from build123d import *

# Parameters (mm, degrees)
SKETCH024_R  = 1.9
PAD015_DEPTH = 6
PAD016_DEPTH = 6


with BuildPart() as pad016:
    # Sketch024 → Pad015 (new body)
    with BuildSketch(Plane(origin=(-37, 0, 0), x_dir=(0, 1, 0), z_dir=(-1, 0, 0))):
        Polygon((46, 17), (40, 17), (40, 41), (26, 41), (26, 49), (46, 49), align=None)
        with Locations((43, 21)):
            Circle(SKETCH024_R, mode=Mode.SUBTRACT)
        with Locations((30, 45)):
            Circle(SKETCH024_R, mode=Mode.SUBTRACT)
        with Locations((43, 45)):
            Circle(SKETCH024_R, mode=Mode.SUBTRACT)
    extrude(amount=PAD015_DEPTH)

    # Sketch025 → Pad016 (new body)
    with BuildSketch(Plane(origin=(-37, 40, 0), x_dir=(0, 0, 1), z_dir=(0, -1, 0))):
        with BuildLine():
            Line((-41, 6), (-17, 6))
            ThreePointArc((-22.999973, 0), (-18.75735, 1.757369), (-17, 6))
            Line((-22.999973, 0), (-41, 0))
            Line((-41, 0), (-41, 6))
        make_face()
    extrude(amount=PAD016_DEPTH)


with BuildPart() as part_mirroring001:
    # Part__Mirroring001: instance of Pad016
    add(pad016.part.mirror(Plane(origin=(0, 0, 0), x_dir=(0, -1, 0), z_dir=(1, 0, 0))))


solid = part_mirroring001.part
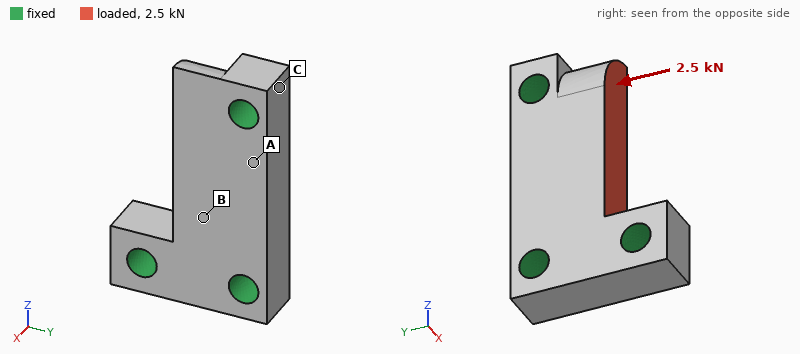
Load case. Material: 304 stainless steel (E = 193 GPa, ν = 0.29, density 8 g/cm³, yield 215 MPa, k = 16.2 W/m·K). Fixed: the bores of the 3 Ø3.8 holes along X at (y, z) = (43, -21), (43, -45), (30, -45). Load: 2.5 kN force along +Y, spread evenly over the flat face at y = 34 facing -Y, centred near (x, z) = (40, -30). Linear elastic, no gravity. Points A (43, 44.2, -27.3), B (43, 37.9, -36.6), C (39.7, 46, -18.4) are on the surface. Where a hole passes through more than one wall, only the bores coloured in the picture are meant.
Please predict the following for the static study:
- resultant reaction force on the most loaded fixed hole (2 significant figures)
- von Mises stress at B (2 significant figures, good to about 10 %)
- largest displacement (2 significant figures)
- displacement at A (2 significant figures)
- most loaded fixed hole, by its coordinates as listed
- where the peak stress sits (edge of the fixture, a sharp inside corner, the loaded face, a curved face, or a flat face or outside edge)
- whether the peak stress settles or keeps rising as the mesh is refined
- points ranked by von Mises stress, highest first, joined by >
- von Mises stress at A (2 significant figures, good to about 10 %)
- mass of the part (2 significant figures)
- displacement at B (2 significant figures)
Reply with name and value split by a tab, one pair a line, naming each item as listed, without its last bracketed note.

resultant reaction force on the most loaded fixed hole	1.5 kN
von Mises stress at B	22 MPa
largest displacement	2.3 µm
displacement at A	1.4 µm
most loaded fixed hole, by its coordinates as listed	(43, -21)
where the peak stress sits	edge of the fixture
whether the peak stress settles or keeps rising as the mesh is refined	keeps rising
points ranked by von Mises stress, highest first, joined by >	B > A > C
von Mises stress at A	12 MPa
mass of the part	20 g
displacement at B	1.7 µm
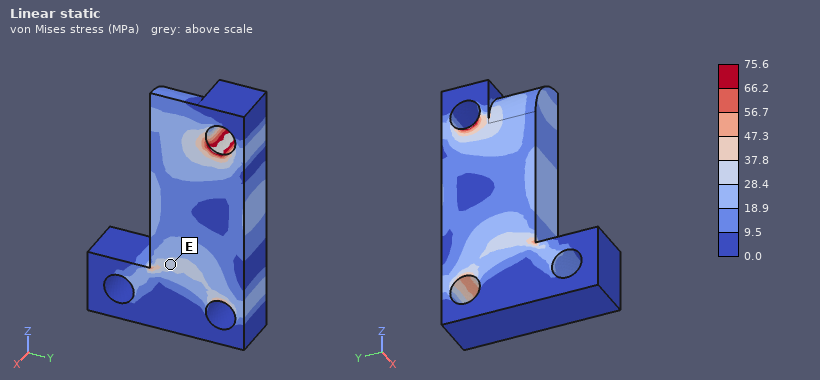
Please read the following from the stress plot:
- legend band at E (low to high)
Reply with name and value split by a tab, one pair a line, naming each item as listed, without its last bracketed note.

legend band at E	28.4 to 37.8 MPa
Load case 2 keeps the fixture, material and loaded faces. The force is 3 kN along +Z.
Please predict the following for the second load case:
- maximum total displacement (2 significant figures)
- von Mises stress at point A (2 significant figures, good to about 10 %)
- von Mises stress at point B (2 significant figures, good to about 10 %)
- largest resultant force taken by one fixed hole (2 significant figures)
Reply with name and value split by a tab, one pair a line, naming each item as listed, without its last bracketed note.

maximum total displacement	5.2 µm
von Mises stress at point A	13 MPa
von Mises stress at point B	33 MPa
largest resultant force taken by one fixed hole	1.6 kN
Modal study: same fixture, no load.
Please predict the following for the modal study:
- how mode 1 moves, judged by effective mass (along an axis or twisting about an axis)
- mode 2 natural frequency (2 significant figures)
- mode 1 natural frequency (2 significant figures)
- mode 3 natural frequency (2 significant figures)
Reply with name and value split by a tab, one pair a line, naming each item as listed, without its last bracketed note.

how mode 1 moves, judged by effective mass	along X
mode 2 natural frequency	52 kHz
mode 1 natural frequency	37 kHz
mode 3 natural frequency	52 kHz
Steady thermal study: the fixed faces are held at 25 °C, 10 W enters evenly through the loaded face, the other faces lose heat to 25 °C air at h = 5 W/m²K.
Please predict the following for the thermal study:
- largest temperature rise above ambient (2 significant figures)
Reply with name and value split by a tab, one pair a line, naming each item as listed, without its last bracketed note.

largest temperature rise above ambient	48 K
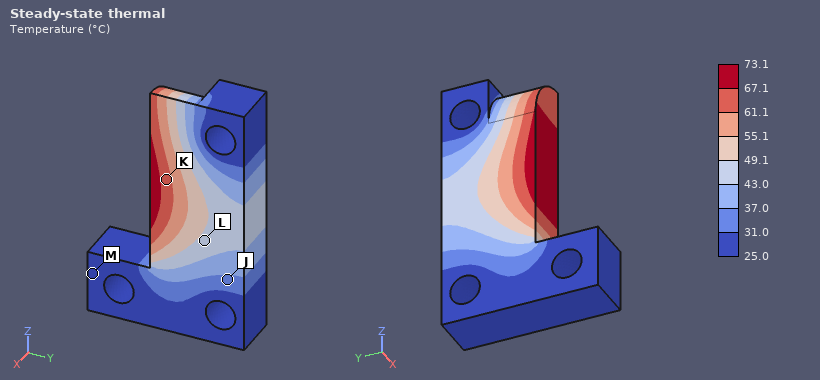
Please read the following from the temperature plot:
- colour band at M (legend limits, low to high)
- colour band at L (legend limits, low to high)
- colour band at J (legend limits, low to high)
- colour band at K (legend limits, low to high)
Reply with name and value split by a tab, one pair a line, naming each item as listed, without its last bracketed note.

colour band at M	25.0 to 31.0 °C
colour band at L	43.0 to 49.1 °C
colour band at J	31.0 to 37.0 °C
colour band at K	61.1 to 67.1 °C
